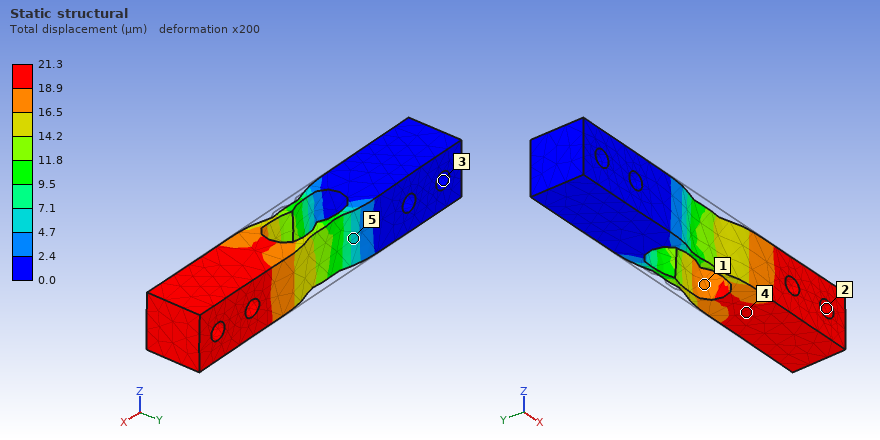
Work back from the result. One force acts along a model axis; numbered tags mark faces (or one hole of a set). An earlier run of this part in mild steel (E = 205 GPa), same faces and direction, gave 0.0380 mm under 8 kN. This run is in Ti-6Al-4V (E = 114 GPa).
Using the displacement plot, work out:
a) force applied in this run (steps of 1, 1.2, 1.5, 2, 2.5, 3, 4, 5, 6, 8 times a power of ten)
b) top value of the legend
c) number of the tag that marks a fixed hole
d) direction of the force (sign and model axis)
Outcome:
2.5 kN
21.3 µm
3
+X
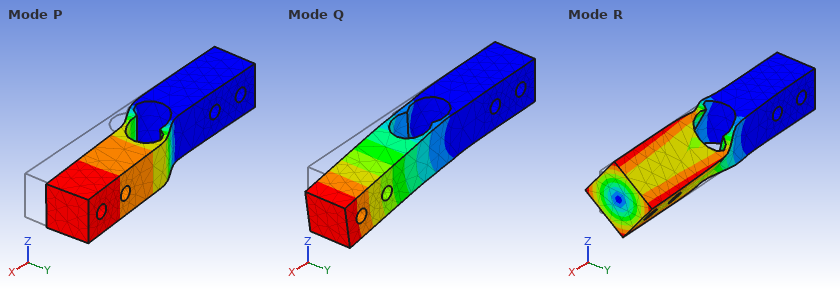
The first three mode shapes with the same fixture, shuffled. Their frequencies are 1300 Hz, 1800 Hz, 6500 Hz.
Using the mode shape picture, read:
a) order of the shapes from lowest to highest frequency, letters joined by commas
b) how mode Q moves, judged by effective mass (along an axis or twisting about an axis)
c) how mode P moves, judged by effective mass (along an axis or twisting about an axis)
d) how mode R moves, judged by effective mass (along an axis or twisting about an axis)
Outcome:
P, Q, R
along Z
along Y
twisting about X
